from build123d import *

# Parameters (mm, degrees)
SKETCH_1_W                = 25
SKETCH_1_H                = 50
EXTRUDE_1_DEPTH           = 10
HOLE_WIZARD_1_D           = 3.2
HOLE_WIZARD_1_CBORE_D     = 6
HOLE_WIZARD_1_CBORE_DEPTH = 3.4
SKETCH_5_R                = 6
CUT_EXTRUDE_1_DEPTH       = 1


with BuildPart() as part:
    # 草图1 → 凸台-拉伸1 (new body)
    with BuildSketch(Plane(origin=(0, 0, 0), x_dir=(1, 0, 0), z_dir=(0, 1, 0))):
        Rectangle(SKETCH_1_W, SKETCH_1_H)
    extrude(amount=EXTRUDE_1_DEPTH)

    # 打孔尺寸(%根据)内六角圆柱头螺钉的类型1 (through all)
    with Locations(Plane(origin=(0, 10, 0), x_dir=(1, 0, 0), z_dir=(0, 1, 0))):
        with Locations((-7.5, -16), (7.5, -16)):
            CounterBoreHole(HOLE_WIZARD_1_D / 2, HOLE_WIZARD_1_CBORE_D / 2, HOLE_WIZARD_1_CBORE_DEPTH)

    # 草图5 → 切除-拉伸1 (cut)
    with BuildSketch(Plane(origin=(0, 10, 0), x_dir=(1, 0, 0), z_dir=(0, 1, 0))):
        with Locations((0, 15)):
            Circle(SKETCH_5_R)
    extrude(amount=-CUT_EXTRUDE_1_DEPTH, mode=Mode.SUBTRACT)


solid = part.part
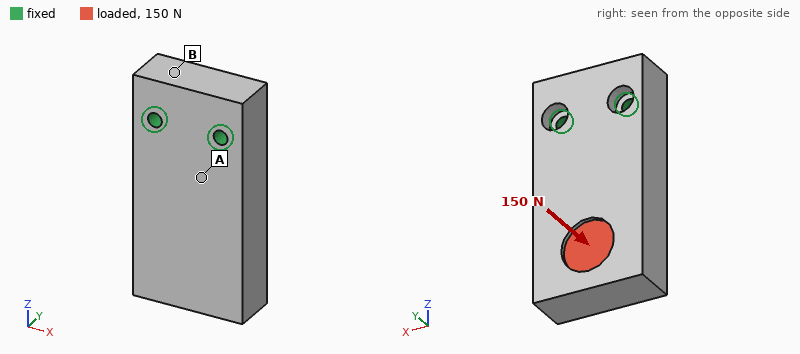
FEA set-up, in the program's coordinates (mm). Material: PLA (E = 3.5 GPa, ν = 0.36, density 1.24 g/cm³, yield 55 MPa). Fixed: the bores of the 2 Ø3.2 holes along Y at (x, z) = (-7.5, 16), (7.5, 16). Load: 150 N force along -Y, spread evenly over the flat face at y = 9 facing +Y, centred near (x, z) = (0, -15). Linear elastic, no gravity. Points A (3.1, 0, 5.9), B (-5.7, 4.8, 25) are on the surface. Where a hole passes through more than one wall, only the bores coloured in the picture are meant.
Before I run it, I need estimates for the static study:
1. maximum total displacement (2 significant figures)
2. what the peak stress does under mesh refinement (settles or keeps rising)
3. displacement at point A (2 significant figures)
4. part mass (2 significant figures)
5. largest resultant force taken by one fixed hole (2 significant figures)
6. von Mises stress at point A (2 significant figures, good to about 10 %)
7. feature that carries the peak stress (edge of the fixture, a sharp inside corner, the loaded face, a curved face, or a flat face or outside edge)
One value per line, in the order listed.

0.51 mm
keeps rising
0.089 mm
15 g
80 N
7.3 MPa
edge of the fixture
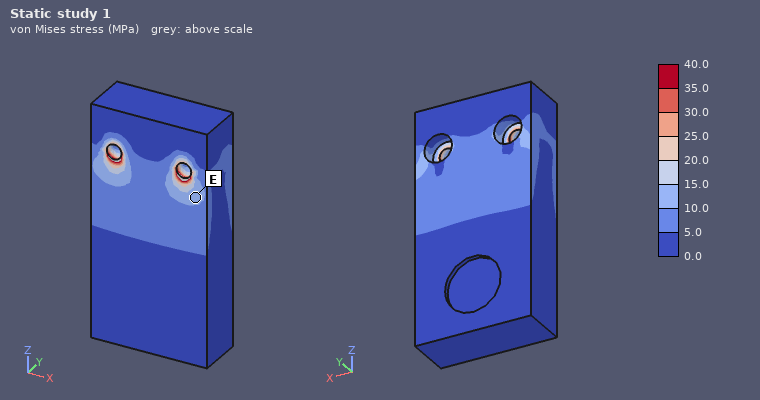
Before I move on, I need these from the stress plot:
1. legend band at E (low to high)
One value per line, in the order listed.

10.0 to 15.0 MPa
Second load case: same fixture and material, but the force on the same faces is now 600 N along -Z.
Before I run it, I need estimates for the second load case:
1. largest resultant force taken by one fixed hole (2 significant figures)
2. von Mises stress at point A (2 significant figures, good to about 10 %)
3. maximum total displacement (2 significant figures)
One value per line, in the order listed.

300 N
3.3 MPa
0.43 mm
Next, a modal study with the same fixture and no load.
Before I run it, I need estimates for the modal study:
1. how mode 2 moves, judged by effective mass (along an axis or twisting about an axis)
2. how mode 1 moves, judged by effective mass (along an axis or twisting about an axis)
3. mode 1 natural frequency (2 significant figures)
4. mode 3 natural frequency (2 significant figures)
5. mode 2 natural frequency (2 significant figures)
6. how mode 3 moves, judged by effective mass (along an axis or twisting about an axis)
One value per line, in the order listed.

along X
along Y
1200 Hz
4100 Hz
2900 Hz
twisting about Z
